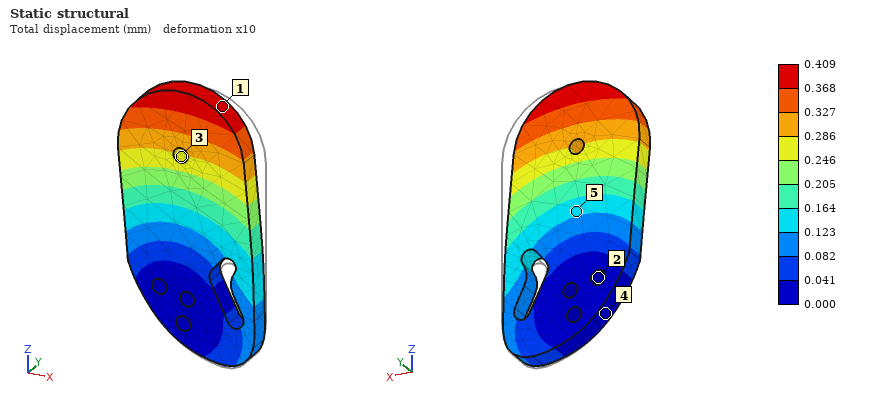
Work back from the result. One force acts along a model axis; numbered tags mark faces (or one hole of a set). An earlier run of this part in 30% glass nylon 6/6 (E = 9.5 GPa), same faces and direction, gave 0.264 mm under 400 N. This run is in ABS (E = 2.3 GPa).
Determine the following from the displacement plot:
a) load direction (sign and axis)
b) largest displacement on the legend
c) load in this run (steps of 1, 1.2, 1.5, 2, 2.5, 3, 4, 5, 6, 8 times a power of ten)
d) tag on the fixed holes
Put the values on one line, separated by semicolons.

-X; 0.409 mm; 150 N; 2
